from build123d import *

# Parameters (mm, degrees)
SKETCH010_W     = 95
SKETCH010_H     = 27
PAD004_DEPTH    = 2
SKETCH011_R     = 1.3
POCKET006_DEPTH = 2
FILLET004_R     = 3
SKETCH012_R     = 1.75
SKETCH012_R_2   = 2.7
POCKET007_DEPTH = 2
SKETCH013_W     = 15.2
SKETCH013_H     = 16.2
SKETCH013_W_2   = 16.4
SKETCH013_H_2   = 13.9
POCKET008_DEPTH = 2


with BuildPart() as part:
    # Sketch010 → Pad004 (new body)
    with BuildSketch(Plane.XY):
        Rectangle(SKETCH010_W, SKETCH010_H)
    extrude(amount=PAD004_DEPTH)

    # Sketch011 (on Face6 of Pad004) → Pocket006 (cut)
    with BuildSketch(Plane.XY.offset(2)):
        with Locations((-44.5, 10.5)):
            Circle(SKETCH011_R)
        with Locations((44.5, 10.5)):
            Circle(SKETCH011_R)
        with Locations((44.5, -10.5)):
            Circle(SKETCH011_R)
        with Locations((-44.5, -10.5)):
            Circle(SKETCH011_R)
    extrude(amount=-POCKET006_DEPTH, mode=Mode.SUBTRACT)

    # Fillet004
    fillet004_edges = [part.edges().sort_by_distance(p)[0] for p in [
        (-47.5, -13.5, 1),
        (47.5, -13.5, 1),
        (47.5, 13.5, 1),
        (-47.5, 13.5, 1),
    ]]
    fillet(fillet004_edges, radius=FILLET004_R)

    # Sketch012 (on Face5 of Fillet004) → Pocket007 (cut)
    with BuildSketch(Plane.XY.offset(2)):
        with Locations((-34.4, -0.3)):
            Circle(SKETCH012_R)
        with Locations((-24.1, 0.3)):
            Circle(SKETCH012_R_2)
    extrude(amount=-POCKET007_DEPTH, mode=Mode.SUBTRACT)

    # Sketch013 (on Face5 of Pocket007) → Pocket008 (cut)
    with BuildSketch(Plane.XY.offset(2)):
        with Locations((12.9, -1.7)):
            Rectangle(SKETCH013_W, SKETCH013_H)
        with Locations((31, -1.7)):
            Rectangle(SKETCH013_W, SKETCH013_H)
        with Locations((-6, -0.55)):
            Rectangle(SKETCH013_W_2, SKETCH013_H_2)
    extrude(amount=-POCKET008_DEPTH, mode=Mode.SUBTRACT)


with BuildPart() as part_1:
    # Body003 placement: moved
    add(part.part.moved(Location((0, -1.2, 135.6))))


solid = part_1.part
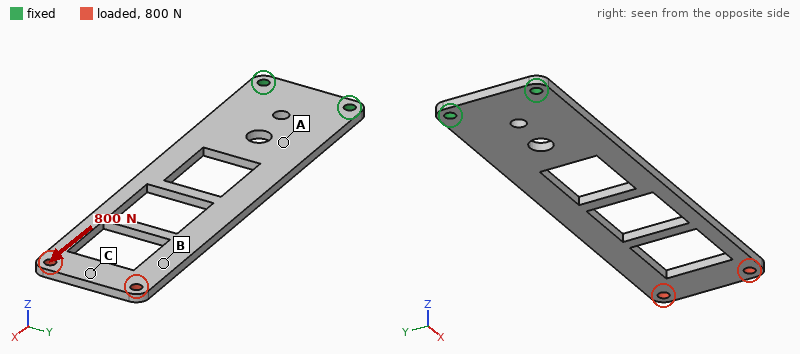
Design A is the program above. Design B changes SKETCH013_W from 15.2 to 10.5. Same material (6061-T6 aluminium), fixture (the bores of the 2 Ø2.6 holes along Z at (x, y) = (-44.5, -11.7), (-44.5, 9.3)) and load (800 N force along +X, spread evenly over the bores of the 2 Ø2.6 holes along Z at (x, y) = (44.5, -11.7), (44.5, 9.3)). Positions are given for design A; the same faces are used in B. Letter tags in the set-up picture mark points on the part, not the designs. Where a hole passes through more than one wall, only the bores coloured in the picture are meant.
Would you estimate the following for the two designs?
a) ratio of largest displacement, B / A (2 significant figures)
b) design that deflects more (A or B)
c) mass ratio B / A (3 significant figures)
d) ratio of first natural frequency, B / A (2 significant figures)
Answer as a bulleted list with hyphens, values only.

- 0.89
- A
- 1.09
- 0.93
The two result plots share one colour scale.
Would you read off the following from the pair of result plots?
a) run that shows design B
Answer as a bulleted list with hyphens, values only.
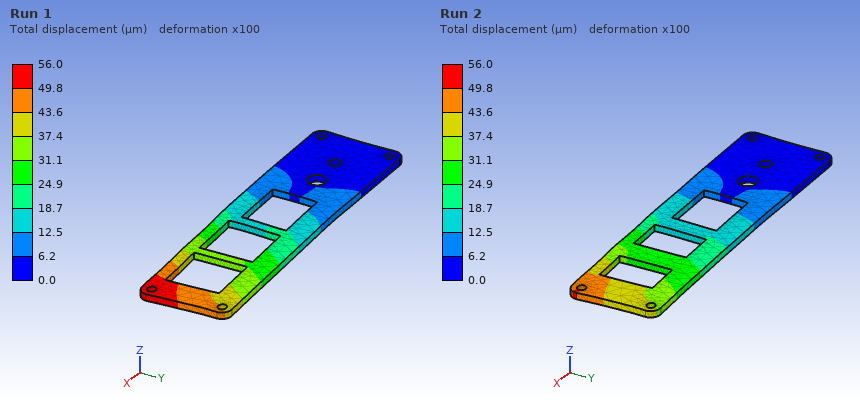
- Run 2
